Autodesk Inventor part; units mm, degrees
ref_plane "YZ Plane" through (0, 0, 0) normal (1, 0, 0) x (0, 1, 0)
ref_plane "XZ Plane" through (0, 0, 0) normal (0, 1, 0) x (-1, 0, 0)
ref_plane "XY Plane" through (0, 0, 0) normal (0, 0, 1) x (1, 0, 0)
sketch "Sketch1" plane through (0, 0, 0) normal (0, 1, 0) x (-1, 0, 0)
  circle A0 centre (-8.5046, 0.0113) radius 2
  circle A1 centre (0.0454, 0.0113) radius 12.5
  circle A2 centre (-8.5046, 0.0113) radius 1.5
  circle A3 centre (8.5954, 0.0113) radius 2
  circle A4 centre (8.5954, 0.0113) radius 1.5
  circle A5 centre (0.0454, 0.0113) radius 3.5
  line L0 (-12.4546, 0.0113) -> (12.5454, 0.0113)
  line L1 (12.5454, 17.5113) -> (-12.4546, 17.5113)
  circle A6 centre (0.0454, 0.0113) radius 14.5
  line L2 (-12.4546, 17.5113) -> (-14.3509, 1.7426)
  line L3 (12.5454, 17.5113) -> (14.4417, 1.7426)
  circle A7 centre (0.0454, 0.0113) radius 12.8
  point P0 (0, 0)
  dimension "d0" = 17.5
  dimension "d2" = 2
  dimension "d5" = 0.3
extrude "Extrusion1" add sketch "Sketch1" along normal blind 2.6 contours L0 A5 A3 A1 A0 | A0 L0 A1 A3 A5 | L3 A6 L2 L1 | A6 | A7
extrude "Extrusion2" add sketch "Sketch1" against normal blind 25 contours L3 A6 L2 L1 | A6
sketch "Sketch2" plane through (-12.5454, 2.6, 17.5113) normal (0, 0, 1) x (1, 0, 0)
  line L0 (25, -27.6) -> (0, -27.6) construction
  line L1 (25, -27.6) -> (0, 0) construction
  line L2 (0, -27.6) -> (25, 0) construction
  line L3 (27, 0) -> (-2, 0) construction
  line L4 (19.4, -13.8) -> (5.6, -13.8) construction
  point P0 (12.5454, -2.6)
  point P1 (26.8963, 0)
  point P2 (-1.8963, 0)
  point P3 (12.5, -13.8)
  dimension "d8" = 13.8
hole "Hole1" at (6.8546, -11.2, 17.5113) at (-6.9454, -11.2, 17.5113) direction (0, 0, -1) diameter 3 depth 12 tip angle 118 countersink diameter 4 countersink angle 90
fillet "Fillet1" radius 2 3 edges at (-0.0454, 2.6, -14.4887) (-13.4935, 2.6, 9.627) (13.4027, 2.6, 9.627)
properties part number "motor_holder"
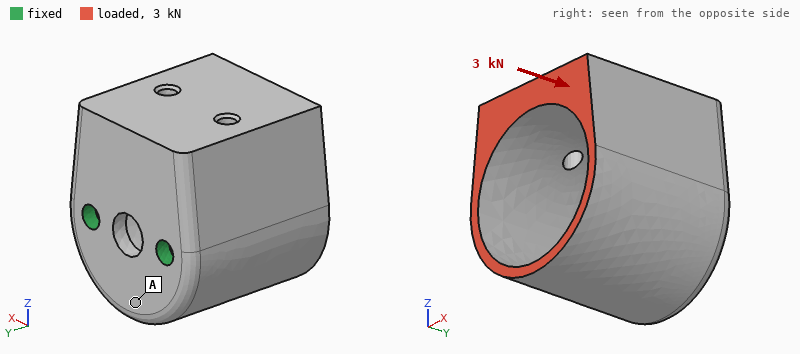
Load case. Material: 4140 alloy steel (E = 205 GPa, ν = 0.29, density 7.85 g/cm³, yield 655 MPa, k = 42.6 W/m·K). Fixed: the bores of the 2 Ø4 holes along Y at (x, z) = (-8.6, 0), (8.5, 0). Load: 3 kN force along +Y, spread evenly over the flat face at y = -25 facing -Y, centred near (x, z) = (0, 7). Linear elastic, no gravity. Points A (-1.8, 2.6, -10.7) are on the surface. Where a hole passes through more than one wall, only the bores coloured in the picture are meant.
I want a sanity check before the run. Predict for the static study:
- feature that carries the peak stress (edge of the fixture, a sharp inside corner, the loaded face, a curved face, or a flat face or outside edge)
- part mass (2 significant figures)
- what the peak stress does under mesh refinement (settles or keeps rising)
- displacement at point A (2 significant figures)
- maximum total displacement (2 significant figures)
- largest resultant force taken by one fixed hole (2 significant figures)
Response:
edge of the fixture
71 g
keeps rising
0.020 mm
0.10 mm
1.5 kN
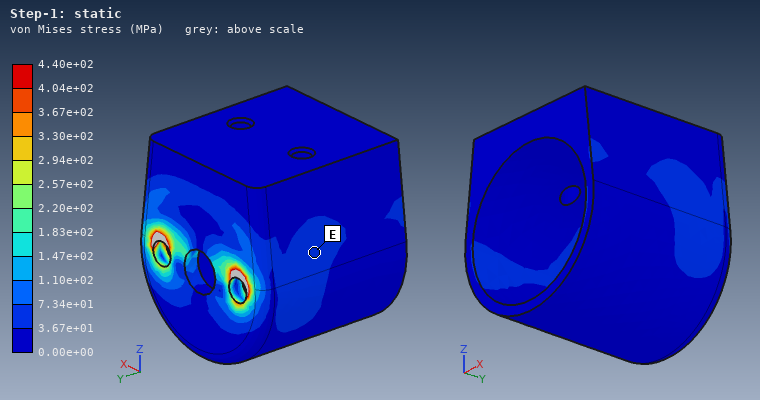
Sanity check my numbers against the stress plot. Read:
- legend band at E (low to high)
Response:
3.67e+01 to 7.34e+01 MPa
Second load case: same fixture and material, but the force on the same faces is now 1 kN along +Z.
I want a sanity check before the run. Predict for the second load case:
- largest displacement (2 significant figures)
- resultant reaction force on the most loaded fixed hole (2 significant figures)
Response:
0.13 mm
500 N
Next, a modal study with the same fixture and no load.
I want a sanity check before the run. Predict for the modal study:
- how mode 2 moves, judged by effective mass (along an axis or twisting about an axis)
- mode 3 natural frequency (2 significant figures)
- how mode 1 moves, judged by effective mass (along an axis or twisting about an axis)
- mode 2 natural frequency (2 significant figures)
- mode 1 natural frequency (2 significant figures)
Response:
along X
9700 Hz
along Z
6300 Hz
2700 Hz
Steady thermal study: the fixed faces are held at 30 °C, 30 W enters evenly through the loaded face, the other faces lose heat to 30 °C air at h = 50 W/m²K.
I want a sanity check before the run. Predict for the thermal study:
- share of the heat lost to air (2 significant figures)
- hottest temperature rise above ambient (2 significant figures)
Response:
43 %
83 K
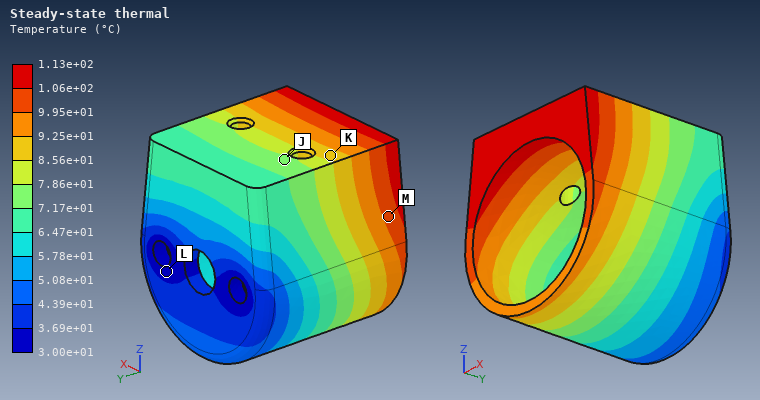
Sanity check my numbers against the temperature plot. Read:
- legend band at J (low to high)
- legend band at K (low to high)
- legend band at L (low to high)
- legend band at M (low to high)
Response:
7.17e+01 to 7.86e+01 °C
8.56e+01 to 9.25e+01 °C
3.00e+01 to 3.69e+01 °C
9.95e+01 to 1.06e+02 °C
